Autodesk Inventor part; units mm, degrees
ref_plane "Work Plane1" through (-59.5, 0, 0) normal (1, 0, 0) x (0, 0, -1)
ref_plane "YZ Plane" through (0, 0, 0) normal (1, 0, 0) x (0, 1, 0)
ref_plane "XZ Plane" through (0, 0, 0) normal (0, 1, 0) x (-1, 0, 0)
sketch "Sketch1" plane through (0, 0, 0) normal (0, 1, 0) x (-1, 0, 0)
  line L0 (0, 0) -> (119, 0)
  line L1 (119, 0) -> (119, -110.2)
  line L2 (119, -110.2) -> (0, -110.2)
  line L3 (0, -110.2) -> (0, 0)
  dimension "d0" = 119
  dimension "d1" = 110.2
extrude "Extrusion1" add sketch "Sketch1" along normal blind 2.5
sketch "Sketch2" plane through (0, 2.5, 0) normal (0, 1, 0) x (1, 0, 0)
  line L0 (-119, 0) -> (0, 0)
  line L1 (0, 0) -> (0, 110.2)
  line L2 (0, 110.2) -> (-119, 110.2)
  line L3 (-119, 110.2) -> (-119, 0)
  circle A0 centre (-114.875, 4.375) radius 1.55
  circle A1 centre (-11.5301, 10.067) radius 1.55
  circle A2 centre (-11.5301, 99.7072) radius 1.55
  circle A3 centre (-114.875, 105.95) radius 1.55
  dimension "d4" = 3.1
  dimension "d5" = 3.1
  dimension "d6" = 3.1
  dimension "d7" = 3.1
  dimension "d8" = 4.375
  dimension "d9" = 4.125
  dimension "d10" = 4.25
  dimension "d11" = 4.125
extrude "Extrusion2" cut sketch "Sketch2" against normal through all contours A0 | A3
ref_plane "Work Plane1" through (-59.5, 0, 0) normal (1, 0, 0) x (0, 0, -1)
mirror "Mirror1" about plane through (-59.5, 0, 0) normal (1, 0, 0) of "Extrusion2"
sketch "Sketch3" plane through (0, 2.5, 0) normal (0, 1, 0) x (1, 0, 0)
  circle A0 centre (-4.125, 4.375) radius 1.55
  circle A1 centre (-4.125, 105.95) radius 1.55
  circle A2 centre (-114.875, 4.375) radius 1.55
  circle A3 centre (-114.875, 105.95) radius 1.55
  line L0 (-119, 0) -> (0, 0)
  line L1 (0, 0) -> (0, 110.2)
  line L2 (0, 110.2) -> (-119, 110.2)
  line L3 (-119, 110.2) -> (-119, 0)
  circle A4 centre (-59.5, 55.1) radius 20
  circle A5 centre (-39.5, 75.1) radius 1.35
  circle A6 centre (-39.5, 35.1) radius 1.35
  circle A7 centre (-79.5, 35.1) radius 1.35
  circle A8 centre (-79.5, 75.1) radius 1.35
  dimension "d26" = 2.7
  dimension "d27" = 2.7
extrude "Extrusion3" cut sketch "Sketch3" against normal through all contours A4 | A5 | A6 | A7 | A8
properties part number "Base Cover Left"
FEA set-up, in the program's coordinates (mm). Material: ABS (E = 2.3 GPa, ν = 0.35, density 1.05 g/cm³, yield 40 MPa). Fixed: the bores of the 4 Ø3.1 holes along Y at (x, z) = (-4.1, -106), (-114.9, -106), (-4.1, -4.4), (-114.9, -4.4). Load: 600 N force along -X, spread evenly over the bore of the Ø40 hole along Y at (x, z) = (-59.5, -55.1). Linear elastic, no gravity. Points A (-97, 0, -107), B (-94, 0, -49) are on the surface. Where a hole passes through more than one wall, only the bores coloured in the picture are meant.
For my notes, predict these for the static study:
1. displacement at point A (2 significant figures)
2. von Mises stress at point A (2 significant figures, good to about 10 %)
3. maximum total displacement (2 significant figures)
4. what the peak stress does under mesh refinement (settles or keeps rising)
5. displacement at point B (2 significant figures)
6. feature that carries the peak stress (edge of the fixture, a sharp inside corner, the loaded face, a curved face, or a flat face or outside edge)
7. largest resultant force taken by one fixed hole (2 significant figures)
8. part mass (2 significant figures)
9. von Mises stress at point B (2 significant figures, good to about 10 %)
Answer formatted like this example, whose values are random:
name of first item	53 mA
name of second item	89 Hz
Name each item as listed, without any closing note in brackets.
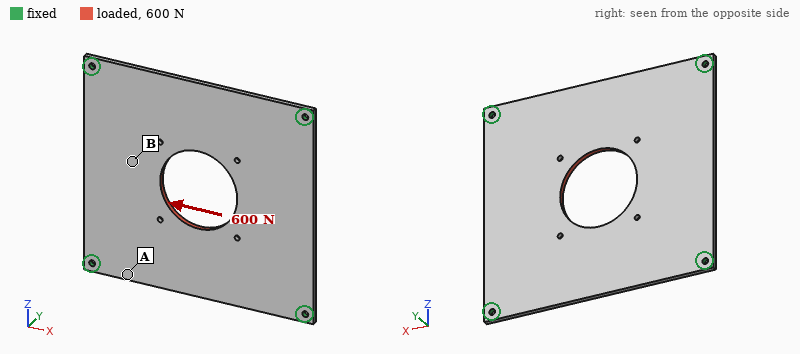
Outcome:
displacement at point A	0.032 mm
von Mises stress at point A	2.8 MPa
maximum total displacement	0.10 mm
what the peak stress does under mesh refinement	keeps rising
displacement at point B	0.091 mm
feature that carries the peak stress	edge of the fixture
largest resultant force taken by one fixed hole	170 N
part mass	31 g
von Mises stress at point B	1.2 MPa
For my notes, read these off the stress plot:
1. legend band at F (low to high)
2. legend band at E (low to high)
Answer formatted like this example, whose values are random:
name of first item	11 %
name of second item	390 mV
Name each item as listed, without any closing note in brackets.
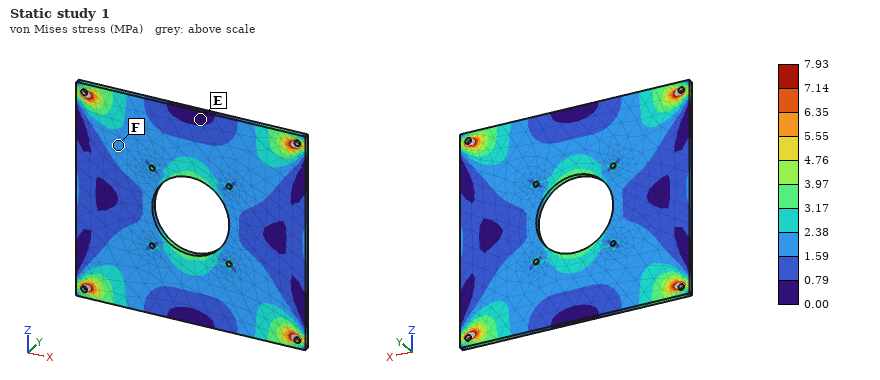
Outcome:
legend band at F	1.59 to 2.38 MPa
legend band at E	0.00 to 0.79 MPa
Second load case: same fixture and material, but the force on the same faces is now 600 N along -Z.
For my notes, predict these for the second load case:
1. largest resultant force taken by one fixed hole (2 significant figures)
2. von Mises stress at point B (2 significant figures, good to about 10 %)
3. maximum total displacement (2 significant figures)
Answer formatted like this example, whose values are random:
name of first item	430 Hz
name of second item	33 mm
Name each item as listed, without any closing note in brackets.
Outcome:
largest resultant force taken by one fixed hole	170 N
von Mises stress at point B	2.4 MPa
maximum total displacement	0.11 mm
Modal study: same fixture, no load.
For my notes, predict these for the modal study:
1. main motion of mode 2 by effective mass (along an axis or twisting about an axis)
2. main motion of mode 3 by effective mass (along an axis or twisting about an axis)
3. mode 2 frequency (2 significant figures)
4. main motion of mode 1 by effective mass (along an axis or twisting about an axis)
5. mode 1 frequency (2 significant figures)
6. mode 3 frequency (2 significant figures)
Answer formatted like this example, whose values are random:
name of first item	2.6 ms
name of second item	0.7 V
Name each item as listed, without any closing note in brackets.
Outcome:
main motion of mode 2 by effective mass	twisting about X
main motion of mode 3 by effective mass	twisting about Z
mode 2 frequency	340 Hz
main motion of mode 1 by effective mass	along Y
mode 1 frequency	200 Hz
mode 3 frequency	370 Hz
